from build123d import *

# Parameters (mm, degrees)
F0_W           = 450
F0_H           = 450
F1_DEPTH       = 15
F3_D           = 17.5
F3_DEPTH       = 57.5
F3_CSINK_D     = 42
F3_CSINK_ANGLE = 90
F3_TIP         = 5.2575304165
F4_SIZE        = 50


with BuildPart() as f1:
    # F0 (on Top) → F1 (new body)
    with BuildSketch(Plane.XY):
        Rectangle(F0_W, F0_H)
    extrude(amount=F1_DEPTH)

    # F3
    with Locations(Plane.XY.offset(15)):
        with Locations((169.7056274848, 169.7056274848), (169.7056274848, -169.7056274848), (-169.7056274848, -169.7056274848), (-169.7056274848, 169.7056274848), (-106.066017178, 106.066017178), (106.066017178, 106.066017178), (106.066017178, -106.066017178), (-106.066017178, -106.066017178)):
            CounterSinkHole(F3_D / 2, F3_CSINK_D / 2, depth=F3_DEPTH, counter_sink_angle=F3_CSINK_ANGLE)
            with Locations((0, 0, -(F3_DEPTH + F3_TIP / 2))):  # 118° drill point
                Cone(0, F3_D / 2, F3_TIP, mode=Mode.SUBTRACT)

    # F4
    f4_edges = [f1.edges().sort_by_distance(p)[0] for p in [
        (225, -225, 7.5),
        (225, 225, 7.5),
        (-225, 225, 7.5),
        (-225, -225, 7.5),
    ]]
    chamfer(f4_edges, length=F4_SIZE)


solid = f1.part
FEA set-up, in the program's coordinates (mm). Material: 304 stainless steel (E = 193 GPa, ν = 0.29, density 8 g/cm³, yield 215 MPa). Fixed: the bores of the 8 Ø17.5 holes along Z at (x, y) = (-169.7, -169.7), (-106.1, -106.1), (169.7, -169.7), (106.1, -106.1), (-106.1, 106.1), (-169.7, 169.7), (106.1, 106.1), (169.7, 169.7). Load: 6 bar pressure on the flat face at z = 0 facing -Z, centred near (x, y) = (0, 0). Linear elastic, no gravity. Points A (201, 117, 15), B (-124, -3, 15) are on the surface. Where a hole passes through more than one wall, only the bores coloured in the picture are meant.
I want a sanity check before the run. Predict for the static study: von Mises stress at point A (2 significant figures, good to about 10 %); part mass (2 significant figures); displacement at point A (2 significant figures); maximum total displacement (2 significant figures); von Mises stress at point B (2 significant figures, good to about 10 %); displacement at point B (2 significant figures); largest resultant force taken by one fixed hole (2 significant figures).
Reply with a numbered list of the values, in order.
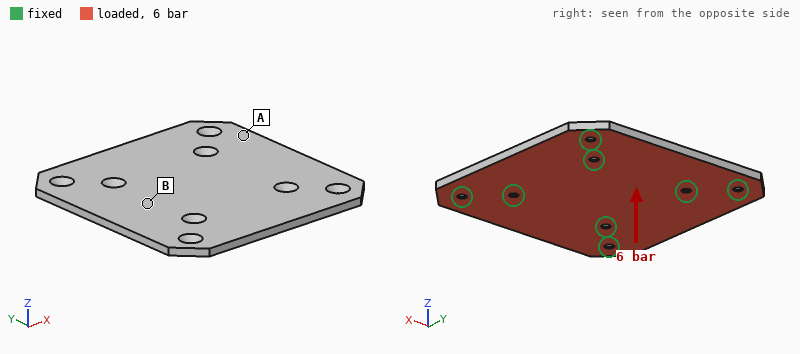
1. 20 MPa
2. 23 kg
3. 0.084 mm
4. 0.26 mm
5. 57 MPa
6. 0.13 mm
7. 23 kN
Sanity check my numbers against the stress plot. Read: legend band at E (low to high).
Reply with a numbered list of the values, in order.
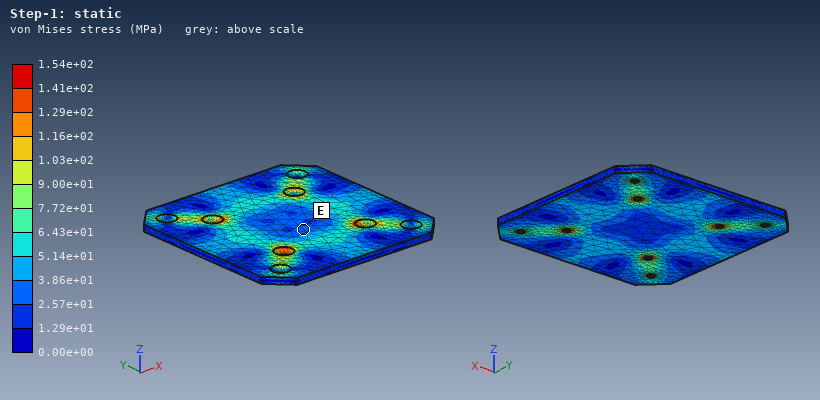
1. 2.57e+01 to 3.86e+01 MPa
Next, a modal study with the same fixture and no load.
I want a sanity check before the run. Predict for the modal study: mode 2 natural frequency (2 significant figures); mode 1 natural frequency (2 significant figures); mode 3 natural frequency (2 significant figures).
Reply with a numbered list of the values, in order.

1. 730 Hz
2. 620 Hz
3. 730 Hz
